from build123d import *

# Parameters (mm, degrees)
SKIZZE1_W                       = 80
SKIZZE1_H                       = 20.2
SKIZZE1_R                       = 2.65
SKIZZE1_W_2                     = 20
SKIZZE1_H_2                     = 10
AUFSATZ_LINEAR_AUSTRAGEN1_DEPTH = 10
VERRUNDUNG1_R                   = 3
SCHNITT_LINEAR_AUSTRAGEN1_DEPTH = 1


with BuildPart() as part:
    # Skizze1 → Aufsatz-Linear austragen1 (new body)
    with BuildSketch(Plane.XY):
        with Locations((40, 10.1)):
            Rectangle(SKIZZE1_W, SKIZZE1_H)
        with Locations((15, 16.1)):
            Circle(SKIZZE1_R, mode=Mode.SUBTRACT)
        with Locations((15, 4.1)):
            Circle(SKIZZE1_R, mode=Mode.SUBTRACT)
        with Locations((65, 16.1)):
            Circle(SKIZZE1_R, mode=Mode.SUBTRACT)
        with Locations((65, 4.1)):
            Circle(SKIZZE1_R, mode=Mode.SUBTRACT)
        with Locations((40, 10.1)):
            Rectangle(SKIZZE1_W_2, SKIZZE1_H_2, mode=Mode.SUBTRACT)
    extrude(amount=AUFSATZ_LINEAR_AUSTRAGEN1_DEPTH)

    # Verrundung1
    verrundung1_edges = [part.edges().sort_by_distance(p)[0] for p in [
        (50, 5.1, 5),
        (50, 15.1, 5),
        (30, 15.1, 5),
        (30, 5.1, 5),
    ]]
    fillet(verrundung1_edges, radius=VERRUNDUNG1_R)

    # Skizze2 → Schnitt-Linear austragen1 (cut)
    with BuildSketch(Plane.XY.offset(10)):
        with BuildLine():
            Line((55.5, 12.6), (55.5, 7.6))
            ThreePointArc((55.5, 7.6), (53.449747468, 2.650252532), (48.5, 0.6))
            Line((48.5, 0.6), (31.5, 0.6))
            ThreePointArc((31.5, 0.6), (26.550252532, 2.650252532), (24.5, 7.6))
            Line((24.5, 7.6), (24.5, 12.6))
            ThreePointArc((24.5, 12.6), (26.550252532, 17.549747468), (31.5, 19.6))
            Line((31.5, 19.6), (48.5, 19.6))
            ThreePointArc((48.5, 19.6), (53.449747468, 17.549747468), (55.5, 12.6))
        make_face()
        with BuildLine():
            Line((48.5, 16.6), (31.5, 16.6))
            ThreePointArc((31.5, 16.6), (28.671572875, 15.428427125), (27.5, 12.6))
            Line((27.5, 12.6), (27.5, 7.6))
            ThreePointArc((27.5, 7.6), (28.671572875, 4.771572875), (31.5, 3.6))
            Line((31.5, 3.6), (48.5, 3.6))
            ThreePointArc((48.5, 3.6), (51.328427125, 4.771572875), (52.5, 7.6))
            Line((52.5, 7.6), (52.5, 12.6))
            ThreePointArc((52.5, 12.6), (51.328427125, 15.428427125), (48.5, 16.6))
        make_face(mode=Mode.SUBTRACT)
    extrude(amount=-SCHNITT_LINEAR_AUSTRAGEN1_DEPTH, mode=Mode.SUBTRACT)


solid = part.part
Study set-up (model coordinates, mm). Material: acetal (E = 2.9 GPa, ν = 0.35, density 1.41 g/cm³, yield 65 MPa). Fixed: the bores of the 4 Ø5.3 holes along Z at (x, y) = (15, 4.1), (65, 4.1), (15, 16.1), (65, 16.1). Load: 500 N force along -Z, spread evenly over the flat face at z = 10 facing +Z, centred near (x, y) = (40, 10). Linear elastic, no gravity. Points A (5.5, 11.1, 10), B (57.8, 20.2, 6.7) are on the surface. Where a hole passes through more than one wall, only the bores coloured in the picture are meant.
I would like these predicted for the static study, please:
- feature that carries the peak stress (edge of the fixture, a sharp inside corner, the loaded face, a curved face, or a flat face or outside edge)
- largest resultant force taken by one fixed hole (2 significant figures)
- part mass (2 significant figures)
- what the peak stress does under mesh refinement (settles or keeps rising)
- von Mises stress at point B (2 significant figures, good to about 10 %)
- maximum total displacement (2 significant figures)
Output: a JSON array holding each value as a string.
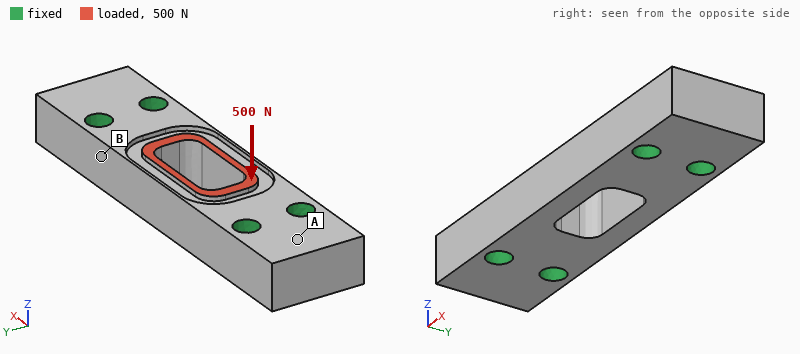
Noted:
["edge of the fixture", "130 N", "18 g", "keeps rising", "3.0 MPa", "86 µm"]
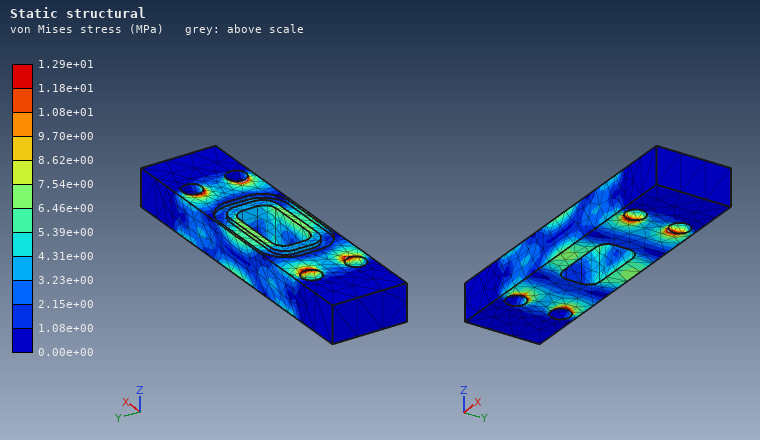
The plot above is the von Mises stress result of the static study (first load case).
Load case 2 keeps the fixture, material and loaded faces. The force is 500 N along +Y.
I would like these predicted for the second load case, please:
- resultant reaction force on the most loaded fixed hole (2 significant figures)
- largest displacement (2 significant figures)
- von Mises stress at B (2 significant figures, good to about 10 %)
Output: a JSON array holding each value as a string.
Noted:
["220 N", "0.12 mm", "4.2 MPa"]
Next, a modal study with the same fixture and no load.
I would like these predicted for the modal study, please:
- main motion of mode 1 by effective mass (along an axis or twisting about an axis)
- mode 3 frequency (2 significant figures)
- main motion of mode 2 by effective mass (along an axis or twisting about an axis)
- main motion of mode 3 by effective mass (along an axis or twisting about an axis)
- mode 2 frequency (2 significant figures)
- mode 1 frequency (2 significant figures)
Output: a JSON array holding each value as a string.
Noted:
["along Z", "8000 Hz", "twisting about X", "along Y", "7500 Hz", "6200 Hz"]
